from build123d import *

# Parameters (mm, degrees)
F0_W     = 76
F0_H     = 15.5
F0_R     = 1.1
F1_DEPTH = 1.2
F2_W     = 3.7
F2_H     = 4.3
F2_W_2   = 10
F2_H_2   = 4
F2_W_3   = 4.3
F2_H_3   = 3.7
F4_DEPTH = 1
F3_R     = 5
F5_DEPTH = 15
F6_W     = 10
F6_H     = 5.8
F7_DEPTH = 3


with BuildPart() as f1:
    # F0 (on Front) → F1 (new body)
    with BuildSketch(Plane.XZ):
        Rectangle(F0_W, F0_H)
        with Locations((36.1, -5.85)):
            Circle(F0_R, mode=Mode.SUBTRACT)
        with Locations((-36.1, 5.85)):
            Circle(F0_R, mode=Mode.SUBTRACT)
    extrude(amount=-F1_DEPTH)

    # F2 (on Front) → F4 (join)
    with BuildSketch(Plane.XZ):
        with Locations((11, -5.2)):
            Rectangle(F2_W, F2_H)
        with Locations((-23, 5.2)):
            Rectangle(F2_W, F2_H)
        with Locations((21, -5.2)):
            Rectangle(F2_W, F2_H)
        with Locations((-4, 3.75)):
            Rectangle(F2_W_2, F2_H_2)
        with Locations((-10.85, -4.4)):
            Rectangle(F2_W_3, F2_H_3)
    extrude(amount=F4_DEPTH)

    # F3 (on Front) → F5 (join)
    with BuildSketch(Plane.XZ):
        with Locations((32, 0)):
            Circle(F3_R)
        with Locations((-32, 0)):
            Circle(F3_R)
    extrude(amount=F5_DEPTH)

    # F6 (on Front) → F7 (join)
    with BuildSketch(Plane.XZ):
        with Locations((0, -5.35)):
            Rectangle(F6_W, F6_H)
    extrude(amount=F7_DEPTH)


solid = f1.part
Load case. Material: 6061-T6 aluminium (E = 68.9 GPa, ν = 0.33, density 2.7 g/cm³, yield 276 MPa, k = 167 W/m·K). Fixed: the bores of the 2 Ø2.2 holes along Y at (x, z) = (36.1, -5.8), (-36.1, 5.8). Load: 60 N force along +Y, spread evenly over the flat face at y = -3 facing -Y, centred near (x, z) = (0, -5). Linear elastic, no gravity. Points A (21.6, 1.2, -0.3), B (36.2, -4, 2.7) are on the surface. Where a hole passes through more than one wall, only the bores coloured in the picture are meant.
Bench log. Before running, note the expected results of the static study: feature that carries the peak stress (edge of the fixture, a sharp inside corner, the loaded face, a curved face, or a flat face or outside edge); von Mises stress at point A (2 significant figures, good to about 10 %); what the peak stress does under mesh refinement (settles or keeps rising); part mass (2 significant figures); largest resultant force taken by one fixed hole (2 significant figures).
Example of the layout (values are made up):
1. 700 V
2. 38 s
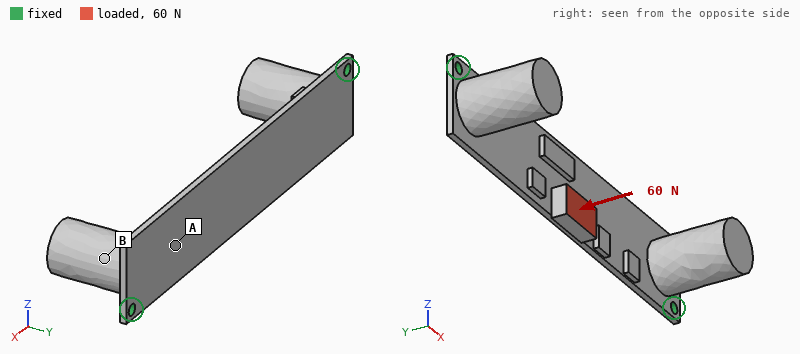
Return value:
1. edge of the fixture
2. 58 MPa
3. keeps rising
4. 11 g
5. 32 N
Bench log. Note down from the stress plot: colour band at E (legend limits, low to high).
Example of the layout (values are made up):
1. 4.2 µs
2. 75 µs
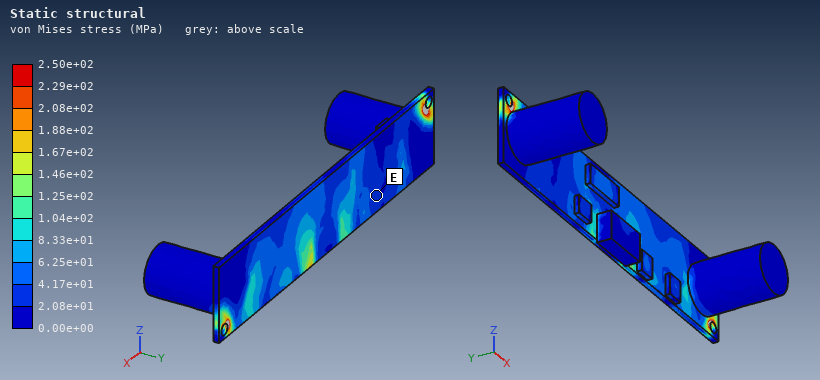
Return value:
1. 2.08e+01 to 4.17e+01 MPa
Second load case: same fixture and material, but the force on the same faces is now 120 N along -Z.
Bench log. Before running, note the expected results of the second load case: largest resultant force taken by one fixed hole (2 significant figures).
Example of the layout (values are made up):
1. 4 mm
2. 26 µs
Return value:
1. 61 N
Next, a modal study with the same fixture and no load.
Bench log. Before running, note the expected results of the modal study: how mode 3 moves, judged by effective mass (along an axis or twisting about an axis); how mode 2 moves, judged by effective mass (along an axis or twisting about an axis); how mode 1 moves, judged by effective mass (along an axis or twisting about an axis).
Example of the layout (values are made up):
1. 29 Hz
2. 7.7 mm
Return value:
1. twisting about Y
2. along Z
3. along Y
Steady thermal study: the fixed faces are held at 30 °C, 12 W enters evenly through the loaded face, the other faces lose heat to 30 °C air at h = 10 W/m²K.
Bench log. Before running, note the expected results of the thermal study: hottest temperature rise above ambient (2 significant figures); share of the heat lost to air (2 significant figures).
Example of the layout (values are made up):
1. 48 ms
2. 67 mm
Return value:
1. 71 K
2. 8.8 %
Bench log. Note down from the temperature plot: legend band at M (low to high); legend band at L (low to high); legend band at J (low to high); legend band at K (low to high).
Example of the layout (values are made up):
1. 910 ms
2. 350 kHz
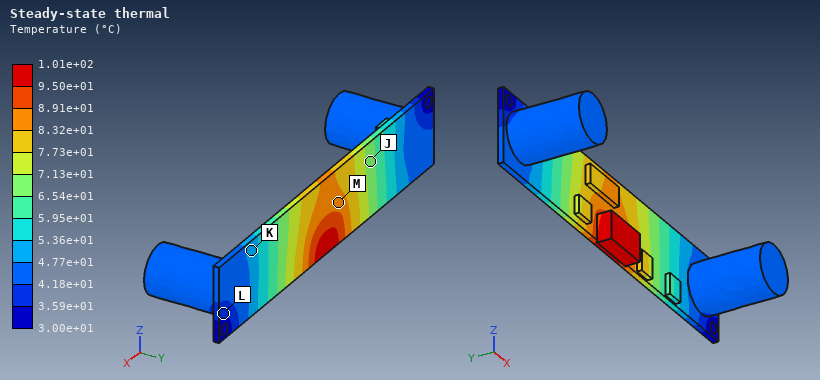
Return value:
1. 8.32e+01 to 8.91e+01 °C
2. 3.59e+01 to 4.18e+01 °C
3. 6.54e+01 to 7.13e+01 °C
4. 4.77e+01 to 5.36e+01 °C
